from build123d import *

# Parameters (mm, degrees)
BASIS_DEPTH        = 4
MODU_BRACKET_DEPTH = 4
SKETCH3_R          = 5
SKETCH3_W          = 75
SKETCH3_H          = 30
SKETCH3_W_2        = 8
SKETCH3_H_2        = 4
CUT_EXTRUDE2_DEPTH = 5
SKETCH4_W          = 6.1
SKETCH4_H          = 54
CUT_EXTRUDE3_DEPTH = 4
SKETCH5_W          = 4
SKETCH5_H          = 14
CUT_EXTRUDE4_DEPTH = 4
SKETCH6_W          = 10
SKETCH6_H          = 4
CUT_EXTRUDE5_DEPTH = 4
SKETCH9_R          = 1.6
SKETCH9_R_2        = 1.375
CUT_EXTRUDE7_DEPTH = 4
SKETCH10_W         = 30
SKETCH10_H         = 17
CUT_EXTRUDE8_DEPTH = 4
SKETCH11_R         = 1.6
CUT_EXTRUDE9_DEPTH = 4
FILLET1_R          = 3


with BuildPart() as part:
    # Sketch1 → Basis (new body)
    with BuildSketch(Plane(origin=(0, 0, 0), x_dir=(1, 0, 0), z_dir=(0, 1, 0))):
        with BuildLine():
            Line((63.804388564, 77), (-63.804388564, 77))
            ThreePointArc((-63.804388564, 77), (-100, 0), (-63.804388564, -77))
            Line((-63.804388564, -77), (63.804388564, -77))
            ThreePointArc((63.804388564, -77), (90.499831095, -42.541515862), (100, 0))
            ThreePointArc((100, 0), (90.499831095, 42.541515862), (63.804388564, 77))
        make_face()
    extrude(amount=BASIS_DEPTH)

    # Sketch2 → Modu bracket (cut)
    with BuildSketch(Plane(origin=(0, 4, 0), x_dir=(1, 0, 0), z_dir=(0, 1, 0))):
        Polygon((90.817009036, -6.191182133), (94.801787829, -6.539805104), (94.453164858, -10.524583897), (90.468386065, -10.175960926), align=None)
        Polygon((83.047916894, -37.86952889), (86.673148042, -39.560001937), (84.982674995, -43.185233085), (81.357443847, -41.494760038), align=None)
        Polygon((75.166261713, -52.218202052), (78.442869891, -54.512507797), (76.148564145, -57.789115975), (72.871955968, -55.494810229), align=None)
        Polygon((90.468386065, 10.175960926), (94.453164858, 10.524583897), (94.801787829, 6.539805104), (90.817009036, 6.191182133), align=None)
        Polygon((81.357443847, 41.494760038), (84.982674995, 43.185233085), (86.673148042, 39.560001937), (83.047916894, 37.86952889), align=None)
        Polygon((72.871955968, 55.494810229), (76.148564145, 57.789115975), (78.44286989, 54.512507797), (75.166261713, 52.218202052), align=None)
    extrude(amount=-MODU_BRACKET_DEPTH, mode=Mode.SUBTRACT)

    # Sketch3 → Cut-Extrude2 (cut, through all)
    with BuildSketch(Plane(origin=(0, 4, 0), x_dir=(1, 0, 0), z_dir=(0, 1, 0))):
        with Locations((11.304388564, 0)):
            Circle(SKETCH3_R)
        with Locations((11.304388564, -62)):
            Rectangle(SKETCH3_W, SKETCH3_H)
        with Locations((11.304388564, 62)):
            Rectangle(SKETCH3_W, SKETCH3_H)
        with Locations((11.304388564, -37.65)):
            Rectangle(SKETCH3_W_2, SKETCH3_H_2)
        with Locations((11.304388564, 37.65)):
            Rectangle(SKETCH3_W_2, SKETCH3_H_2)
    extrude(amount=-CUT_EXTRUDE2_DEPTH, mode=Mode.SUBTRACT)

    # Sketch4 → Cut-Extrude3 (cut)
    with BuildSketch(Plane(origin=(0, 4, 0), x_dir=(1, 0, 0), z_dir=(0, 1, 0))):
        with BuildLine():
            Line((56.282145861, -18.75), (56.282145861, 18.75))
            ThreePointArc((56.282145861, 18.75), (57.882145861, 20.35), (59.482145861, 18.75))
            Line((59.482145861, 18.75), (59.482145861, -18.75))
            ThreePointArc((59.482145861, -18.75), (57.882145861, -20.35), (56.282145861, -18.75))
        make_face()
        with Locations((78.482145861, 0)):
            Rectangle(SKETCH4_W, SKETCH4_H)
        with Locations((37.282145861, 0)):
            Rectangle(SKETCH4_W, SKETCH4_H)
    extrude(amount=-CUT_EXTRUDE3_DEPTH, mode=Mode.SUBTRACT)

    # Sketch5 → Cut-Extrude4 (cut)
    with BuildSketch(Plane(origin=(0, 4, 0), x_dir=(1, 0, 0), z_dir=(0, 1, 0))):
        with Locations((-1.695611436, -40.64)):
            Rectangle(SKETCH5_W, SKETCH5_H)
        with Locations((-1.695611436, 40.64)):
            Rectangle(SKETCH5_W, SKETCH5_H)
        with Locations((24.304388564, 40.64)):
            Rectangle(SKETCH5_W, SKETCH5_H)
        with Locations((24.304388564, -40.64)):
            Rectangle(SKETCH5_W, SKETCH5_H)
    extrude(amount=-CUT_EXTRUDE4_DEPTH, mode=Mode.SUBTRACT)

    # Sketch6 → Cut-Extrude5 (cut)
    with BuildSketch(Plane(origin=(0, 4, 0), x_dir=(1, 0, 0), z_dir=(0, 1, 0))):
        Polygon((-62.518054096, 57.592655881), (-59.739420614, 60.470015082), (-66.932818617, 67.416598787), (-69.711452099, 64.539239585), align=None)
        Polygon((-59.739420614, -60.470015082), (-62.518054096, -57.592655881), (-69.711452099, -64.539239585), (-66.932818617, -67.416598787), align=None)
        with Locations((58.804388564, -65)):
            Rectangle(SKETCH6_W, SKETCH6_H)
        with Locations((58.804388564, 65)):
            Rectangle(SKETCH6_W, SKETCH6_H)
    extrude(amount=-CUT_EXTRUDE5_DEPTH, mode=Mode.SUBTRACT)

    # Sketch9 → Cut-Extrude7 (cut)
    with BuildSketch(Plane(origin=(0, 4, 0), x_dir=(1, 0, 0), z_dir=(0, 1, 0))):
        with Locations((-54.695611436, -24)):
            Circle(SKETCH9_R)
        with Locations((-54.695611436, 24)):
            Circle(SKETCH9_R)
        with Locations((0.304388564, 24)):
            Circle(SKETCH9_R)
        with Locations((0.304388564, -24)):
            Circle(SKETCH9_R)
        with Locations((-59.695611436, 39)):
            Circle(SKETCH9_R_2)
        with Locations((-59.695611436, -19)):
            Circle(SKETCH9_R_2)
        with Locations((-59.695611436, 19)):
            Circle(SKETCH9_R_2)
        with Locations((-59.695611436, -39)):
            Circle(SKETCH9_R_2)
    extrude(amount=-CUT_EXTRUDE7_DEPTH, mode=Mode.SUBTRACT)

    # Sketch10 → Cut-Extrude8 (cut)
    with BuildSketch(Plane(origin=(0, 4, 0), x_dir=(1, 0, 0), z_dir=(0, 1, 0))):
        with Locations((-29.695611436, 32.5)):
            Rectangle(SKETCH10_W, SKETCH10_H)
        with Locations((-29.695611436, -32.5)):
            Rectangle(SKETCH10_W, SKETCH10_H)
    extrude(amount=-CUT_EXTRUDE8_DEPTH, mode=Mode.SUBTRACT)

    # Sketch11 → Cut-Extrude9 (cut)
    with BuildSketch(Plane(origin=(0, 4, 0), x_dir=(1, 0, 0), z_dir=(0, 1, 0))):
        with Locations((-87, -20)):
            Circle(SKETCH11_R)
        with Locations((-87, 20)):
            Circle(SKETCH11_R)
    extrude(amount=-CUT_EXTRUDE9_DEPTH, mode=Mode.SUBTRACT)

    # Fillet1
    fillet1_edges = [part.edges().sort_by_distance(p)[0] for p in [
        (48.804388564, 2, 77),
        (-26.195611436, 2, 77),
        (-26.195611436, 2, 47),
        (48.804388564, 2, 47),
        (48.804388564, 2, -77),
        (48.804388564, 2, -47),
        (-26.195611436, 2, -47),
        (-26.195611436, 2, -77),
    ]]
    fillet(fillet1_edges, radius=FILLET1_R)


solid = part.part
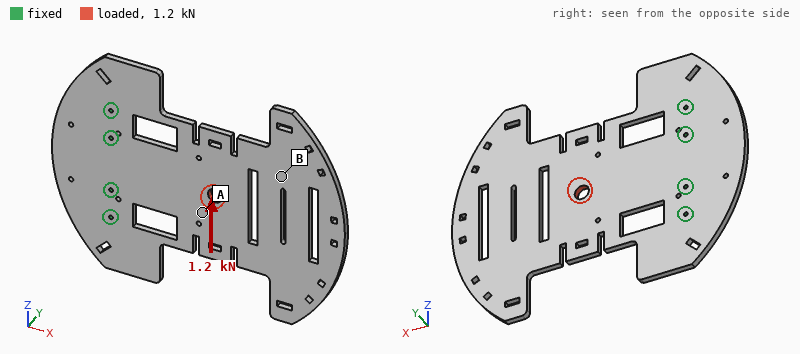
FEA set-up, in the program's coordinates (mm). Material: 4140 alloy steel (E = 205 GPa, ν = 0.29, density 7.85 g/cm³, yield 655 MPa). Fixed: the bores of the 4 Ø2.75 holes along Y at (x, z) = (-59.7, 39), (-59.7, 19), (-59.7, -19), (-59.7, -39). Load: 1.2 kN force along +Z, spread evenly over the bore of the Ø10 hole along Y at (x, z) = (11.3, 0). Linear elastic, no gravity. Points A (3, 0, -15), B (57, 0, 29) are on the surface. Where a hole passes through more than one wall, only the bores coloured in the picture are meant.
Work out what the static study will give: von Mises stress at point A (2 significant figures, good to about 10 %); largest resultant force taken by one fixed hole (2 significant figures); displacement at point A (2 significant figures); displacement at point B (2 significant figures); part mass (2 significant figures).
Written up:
7.6 MPa
860 N
9.0 µm
17 µm
640 g
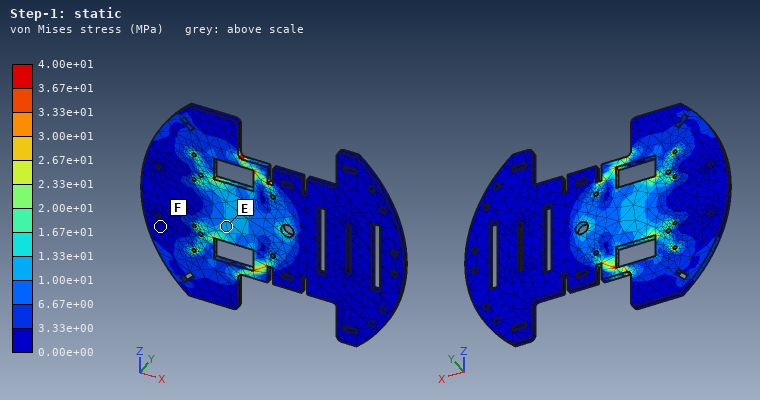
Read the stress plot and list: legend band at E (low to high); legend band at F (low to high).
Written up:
1.00e+01 to 1.33e+01 MPa
0.00e+00 to 3.33e+00 MPa
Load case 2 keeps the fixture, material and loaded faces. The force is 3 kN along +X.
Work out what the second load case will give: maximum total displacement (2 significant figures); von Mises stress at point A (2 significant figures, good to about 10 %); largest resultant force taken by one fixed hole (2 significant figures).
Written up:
6.9 µm
11 MPa
1.1 kN
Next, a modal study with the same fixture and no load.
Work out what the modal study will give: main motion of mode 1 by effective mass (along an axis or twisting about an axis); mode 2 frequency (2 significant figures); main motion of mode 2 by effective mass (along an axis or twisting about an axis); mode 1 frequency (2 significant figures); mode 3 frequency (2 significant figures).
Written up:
along Y
310 Hz
twisting about X
110 Hz
670 Hz
